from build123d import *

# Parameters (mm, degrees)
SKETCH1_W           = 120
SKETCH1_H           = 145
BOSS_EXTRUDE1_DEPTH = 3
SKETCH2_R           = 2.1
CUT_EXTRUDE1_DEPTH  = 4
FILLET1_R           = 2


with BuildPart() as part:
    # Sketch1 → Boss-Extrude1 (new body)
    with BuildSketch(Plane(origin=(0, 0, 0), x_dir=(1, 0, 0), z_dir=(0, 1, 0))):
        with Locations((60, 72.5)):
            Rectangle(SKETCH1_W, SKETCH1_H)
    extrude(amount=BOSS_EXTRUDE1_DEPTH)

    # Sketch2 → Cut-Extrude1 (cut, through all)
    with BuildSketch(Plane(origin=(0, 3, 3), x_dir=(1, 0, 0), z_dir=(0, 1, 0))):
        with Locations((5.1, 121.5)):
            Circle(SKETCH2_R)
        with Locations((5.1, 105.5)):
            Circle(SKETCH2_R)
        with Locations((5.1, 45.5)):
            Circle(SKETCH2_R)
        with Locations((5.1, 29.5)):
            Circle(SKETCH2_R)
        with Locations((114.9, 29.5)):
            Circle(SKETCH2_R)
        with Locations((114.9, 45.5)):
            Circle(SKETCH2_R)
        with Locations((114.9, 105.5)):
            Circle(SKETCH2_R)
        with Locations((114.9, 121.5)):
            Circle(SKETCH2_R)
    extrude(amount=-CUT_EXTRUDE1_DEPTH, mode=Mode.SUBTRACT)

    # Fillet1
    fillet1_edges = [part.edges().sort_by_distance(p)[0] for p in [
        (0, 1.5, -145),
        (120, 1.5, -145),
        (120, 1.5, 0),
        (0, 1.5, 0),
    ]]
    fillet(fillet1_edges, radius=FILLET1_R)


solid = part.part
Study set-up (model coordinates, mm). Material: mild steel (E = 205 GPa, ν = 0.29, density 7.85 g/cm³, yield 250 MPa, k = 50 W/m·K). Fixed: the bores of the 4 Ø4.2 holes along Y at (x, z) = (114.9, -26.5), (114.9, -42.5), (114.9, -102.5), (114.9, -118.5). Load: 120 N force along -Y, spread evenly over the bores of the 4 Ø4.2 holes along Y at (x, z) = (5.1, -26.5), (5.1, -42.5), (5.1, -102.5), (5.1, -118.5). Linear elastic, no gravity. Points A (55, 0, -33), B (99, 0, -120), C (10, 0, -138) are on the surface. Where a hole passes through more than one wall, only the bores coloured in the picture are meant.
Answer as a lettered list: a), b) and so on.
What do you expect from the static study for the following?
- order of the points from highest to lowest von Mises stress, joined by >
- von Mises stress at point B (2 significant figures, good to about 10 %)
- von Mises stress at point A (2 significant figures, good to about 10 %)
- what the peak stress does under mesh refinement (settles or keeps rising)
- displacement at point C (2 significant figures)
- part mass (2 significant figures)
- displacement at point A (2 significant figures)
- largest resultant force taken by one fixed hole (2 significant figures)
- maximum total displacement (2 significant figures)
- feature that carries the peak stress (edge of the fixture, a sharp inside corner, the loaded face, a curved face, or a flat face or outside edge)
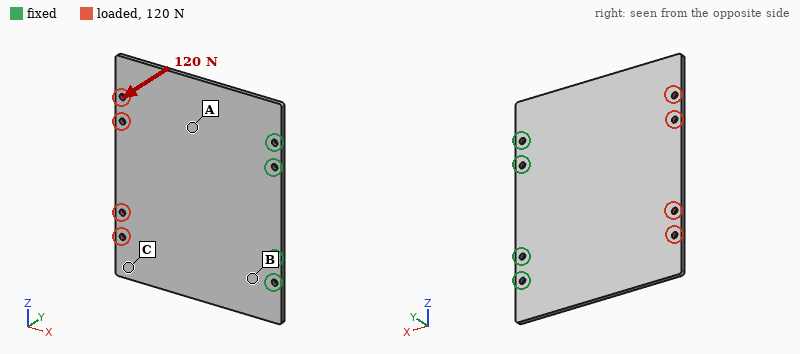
a) B > A > C
b) 53 MPa
c) 26 MPa
d) keeps rising
e) 0.79 mm
f) 410 g
g) 0.33 mm
h) 56 N
i) 0.93 mm
j) edge of the fixture
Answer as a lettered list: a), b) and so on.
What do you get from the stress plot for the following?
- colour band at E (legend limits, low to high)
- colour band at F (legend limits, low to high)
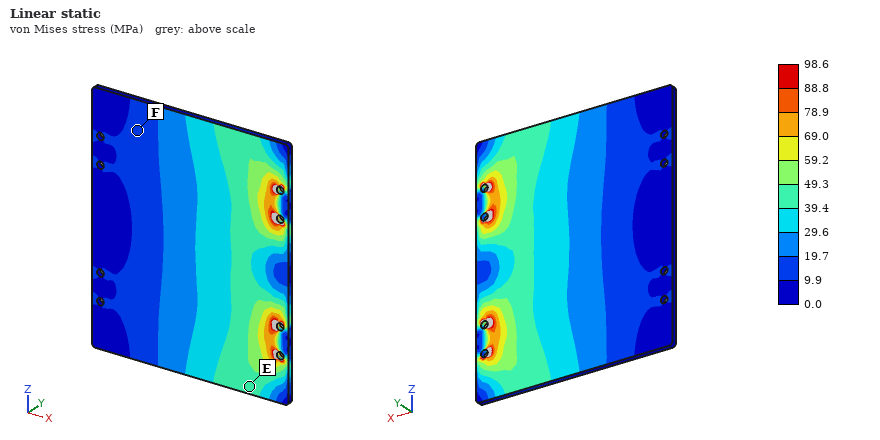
a) 39.4 to 49.3 MPa
b) 9.9 to 19.7 MPa
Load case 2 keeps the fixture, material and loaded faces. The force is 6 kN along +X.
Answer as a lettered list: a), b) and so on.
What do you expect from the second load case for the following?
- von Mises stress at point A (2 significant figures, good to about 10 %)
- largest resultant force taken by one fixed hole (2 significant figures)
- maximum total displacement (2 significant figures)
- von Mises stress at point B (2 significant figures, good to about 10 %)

a) 17 MPa
b) 1.5 kN
c) 13 µm
d) 24 MPa
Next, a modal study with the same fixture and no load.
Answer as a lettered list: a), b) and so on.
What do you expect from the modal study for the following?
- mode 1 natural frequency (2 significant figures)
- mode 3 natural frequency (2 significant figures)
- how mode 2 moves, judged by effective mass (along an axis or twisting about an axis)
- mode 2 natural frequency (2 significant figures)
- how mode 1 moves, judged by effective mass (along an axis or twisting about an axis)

a) 180 Hz
b) 950 Hz
c) twisting about X
d) 380 Hz
e) along Y
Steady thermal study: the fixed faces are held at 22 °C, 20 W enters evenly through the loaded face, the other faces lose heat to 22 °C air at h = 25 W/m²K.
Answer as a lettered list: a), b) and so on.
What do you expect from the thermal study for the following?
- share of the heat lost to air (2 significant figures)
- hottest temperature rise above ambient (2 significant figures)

a) 81 %
b) 59 K
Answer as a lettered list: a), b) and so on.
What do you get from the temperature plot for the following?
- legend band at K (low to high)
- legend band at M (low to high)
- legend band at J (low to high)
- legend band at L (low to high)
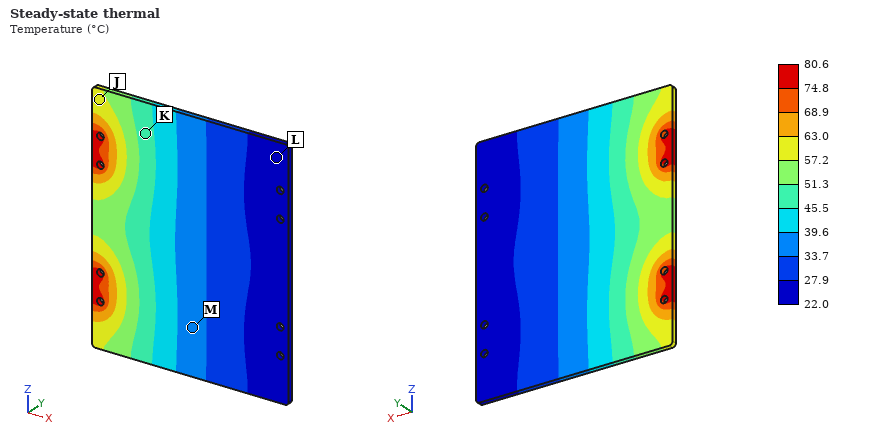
a) 45.5 to 51.3 °C
b) 33.7 to 39.6 °C
c) 57.2 to 63.0 °C
d) 22.0 to 27.9 °C
